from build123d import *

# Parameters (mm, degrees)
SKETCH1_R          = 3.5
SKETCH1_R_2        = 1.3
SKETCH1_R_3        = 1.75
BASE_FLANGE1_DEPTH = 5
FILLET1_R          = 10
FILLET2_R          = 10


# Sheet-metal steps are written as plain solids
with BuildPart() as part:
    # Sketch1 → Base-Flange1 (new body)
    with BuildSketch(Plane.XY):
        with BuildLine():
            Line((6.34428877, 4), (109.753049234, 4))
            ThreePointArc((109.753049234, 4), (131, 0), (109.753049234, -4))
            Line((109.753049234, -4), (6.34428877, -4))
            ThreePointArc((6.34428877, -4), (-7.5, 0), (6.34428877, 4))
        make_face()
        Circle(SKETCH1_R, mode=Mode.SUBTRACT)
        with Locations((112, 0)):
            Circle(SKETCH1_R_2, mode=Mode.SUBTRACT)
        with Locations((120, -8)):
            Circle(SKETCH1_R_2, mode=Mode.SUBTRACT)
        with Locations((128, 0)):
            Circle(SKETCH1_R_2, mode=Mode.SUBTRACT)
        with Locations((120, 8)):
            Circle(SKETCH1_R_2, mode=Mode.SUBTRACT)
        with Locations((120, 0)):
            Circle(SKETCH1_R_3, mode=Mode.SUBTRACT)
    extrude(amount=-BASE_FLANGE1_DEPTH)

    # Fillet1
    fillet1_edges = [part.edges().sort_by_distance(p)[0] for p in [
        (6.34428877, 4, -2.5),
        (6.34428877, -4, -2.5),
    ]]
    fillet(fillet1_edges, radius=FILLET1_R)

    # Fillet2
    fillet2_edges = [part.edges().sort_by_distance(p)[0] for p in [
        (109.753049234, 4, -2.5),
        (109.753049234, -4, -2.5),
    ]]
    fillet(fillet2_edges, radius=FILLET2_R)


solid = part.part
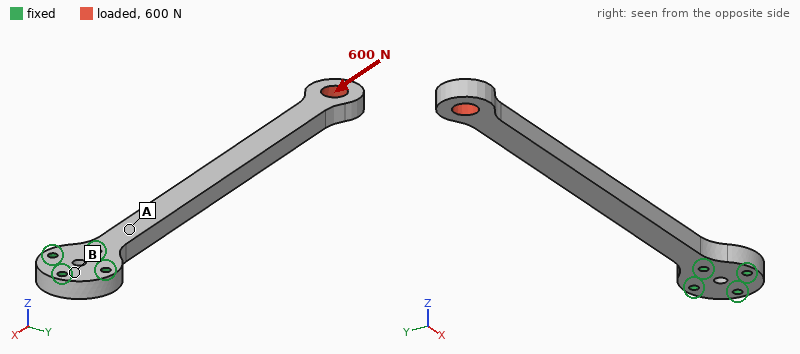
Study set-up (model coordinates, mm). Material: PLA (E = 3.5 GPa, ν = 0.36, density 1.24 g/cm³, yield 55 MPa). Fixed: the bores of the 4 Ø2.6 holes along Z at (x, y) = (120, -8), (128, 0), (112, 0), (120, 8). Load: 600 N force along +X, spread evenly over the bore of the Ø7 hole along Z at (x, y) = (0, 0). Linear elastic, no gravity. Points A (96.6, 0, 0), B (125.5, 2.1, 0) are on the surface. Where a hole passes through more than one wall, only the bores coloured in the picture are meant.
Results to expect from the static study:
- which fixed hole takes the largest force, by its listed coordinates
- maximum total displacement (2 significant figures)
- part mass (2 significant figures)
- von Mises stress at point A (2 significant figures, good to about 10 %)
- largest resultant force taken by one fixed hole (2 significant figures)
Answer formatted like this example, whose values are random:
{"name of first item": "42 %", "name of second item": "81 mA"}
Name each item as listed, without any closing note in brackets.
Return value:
{"which fixed hole takes the largest force, by its listed coordinates": "(112, 0)", "maximum total displacement": "0.52 mm", "part mass": "8.2 g", "von Mises stress at point A": "15 MPa", "largest resultant force taken by one fixed hole": "450 N"}
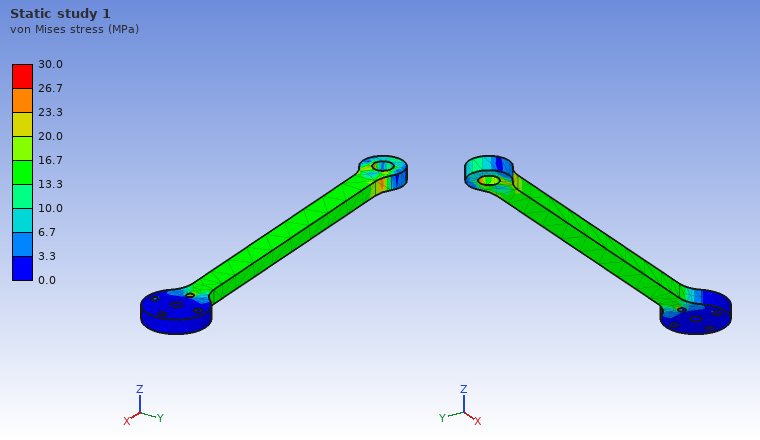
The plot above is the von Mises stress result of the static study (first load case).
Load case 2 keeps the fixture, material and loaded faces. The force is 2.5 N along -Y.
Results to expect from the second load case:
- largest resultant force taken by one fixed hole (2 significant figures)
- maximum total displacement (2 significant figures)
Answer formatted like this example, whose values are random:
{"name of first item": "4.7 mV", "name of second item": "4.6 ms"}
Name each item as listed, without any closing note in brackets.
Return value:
{"largest resultant force taken by one fixed hole": "15 N", "maximum total displacement": "1.7 mm"}
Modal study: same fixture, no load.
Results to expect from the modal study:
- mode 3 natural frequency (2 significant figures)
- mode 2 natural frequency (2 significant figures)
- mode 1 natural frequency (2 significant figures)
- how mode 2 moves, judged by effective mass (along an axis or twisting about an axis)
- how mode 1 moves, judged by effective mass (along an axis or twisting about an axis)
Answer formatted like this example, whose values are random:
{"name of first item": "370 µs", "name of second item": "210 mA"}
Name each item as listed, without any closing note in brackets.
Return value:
{"mode 3 natural frequency": "590 Hz", "mode 2 natural frequency": "150 Hz", "mode 1 natural frequency": "93 Hz", "how mode 2 moves, judged by effective mass": "along Y", "how mode 1 moves, judged by effective mass": "along Z"}
